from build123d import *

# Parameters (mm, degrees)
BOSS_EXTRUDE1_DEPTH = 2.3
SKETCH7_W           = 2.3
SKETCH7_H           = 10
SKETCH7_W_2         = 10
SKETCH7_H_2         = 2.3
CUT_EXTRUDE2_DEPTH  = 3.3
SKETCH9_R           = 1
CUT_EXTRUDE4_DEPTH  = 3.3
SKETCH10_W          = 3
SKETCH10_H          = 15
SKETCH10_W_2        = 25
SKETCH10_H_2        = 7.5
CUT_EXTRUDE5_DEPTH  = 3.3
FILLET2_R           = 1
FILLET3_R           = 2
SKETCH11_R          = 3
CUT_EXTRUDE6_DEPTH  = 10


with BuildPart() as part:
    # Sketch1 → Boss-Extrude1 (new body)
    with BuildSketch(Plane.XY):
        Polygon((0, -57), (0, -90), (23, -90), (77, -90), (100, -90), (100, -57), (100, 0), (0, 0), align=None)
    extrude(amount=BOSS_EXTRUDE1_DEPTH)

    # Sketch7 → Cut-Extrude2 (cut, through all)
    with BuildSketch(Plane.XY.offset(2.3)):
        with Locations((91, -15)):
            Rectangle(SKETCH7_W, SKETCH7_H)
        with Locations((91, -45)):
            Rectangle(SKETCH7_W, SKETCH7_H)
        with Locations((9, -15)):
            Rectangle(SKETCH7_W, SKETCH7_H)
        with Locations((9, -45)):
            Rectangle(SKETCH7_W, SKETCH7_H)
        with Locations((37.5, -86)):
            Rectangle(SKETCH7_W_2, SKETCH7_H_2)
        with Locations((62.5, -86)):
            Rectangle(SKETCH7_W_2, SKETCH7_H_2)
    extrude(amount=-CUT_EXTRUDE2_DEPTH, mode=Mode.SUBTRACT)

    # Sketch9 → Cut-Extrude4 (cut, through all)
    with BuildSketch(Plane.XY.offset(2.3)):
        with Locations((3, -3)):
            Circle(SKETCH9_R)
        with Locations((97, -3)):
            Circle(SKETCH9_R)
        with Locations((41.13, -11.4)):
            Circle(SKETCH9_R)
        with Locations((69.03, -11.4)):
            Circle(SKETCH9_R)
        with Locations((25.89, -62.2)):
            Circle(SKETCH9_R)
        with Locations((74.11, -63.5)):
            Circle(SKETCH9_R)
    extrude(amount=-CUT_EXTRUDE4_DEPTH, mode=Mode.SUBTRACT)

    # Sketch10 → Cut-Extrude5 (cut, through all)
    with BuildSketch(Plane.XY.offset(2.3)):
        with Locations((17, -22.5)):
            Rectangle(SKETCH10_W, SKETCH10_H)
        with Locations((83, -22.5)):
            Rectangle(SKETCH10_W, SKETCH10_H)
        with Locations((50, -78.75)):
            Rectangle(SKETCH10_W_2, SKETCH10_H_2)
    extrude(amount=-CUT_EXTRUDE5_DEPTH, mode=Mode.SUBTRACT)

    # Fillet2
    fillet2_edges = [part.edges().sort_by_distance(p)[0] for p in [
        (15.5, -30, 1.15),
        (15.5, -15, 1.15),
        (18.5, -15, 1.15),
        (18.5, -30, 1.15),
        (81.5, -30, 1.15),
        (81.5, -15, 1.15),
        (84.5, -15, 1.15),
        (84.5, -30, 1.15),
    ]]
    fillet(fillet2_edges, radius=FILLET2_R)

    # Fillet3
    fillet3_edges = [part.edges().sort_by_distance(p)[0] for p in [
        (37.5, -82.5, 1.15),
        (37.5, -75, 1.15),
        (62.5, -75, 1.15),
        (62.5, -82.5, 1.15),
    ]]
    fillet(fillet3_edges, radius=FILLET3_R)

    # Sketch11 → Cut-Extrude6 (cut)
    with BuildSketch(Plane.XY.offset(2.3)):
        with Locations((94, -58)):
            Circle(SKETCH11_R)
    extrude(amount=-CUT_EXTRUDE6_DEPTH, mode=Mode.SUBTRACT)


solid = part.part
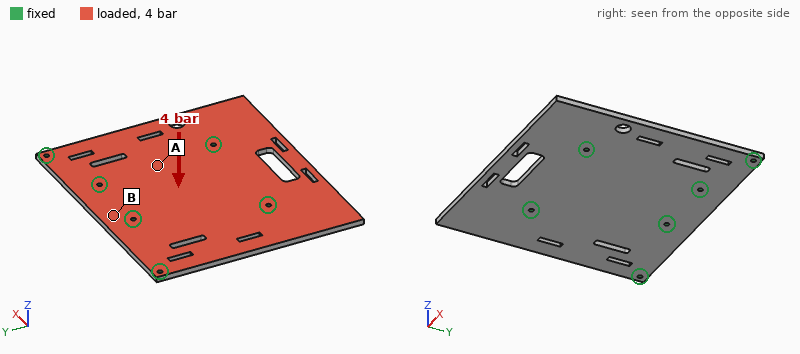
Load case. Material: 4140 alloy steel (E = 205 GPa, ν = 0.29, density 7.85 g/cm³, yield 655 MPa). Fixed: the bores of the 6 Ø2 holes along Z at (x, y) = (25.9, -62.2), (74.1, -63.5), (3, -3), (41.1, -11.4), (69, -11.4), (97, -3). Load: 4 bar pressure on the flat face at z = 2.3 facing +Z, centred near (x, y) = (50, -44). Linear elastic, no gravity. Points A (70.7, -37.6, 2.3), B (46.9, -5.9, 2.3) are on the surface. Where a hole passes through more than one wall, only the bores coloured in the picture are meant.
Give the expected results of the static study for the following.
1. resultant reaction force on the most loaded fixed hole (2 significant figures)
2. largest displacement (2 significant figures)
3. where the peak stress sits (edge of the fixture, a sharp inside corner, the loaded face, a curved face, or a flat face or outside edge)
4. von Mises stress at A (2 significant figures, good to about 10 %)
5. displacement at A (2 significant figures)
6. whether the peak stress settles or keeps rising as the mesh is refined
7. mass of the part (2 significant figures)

1.1 kN
0.29 mm
edge of the fixture
62 MPa
0.048 mm
keeps rising
150 g
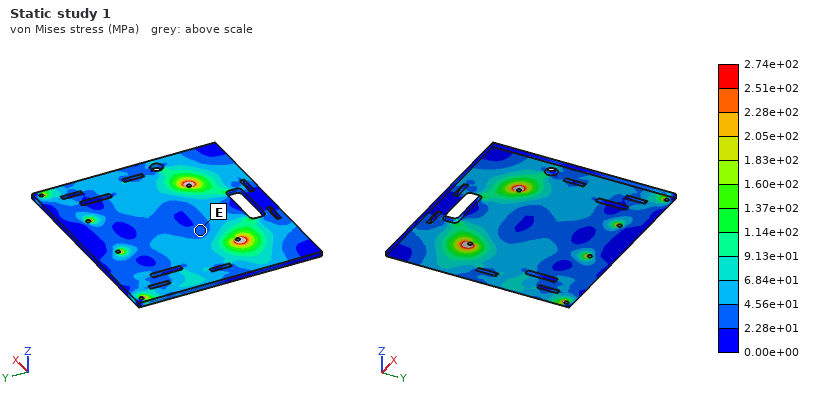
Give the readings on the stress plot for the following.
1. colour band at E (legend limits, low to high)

2.28e+01 to 4.56e+01 MPa
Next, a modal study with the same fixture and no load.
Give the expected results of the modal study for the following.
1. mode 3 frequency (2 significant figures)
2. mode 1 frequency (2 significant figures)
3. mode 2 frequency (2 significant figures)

2200 Hz
1800 Hz
1900 Hz
